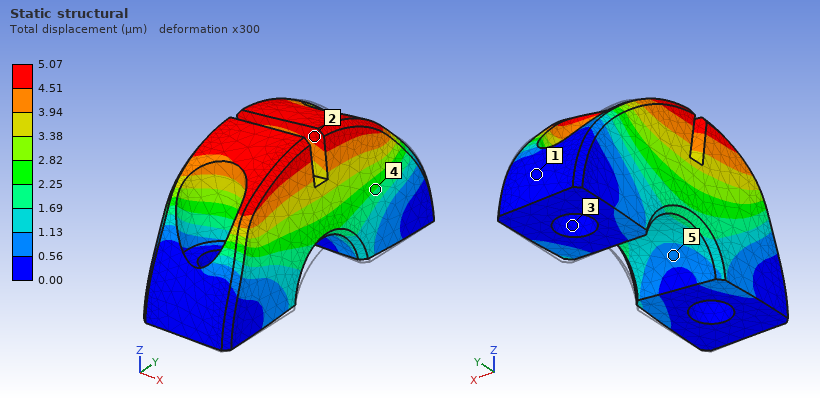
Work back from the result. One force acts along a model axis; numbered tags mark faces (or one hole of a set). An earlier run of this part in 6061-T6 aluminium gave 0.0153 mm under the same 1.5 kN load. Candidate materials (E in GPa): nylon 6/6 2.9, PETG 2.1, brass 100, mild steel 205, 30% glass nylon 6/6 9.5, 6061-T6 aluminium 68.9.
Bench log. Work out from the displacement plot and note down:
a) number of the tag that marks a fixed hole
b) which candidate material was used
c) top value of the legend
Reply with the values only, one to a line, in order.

3
mild steel
5.07 µm
